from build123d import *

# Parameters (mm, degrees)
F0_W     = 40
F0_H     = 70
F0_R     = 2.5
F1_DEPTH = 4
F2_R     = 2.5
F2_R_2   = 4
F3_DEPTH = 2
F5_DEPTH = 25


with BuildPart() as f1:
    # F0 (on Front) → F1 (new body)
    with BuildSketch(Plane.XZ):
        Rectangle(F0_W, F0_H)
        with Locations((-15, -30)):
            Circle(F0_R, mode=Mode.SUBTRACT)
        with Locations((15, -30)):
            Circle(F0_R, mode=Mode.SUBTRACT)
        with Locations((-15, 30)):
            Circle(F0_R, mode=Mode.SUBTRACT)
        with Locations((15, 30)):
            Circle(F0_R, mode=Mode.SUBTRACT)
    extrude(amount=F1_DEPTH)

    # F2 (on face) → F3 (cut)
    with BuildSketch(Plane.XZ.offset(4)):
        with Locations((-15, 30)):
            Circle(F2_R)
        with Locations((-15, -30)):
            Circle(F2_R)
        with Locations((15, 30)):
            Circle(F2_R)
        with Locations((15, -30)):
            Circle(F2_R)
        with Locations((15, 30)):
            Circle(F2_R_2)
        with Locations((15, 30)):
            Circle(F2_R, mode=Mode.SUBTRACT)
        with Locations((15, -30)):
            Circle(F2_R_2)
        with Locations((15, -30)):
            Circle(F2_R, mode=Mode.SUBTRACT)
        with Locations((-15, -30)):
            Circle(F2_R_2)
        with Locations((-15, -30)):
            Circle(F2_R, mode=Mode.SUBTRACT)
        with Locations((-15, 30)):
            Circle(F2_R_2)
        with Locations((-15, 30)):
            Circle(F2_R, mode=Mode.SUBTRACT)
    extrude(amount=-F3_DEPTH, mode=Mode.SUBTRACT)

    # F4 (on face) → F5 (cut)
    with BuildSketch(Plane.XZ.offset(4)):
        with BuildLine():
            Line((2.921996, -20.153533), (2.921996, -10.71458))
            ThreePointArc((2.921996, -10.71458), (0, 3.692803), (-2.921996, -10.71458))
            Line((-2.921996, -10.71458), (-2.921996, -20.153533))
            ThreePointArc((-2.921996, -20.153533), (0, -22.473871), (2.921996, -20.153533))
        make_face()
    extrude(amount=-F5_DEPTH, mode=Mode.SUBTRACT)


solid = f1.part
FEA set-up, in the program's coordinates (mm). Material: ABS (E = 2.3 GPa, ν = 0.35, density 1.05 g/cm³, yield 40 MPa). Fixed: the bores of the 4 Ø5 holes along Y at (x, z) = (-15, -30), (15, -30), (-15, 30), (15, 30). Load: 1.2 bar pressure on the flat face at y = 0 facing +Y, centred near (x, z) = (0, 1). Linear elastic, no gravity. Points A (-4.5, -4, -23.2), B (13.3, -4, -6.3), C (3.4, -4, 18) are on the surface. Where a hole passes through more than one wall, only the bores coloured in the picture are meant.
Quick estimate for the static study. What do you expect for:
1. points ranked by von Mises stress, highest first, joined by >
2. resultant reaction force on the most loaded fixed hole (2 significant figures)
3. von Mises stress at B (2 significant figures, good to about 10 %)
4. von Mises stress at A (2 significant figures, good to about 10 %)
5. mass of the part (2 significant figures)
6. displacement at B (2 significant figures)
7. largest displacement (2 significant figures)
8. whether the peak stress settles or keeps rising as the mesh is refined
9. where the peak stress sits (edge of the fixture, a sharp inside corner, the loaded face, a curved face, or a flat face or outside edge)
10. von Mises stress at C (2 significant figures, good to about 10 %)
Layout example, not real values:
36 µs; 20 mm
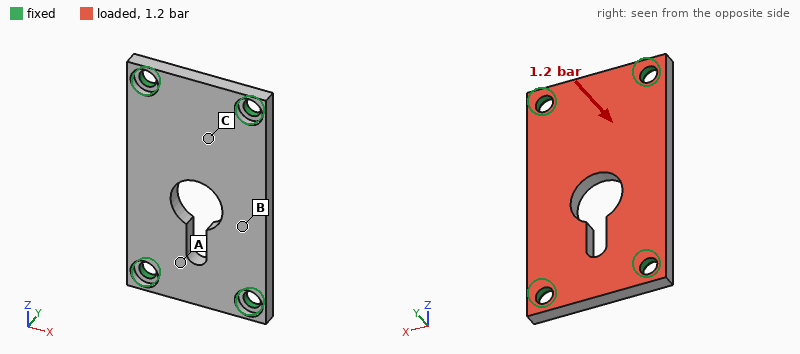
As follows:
B > A > C; 110 N; 9.4 MPa; 5.0 MPa; 10 g; 0.46 mm; 0.53 mm; keeps rising; edge of the fixture; 2.7 MPa
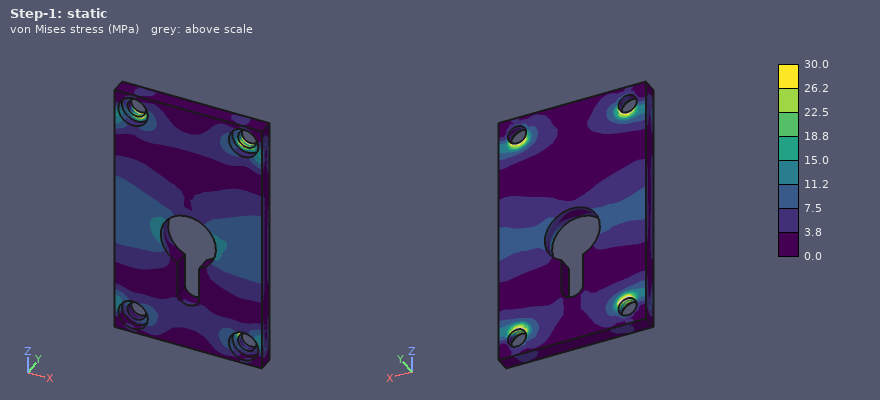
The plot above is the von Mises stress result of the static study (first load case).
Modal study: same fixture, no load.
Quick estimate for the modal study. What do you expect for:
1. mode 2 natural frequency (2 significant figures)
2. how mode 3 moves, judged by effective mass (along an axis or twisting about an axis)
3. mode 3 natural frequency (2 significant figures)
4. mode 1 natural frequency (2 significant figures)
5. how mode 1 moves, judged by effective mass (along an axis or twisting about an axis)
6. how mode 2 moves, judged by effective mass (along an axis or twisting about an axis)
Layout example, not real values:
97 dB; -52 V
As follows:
2000 Hz; twisting about X; 3600 Hz; 1400 Hz; along Y; twisting about Z
